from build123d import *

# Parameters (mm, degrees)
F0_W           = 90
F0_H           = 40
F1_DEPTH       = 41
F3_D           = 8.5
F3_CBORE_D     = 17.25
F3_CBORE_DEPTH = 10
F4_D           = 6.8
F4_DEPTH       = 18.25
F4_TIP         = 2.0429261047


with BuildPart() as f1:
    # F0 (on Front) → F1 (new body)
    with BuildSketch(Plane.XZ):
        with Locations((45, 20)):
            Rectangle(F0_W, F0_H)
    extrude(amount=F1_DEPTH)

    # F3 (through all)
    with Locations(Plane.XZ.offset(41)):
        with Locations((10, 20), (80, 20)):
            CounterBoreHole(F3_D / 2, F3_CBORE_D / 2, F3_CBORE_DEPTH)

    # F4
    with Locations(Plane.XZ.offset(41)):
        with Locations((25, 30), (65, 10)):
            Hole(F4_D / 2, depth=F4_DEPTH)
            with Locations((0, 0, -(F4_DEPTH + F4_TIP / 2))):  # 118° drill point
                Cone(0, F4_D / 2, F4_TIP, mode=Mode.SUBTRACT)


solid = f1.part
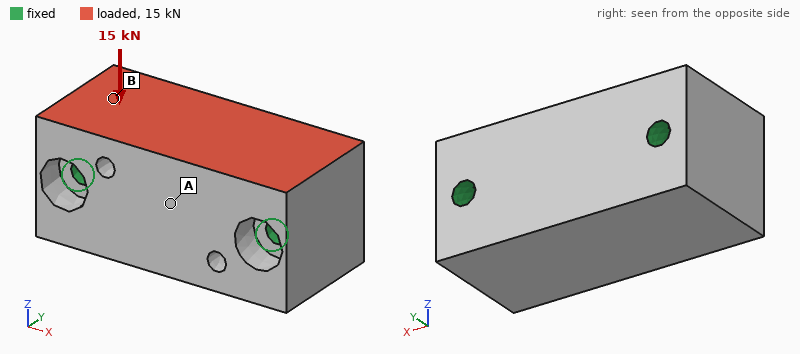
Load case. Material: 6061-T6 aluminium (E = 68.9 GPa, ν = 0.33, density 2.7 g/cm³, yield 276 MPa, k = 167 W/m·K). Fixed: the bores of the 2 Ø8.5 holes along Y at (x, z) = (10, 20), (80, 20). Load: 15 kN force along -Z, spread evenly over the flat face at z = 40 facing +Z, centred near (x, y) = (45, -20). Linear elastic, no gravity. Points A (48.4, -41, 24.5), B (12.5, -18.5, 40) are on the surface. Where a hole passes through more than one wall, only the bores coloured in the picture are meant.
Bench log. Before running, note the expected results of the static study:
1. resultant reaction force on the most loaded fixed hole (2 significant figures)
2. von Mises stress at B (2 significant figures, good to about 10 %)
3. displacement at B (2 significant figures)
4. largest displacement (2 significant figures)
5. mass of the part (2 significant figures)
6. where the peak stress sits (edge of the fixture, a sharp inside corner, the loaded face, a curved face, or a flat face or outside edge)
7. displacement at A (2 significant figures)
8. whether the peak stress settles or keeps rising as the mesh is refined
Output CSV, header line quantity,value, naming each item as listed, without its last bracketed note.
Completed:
quantity,value
resultant reaction force on the most loaded fixed hole,7.5 kN
von Mises stress at B,7.6 MPa
displacement at B,2.9 µm
largest displacement,8.9 µm
mass of the part,370 g
where the peak stress sits,edge of the fixture
displacement at A,7.9 µm
whether the peak stress settles or keeps rising as the mesh is refined,keeps rising
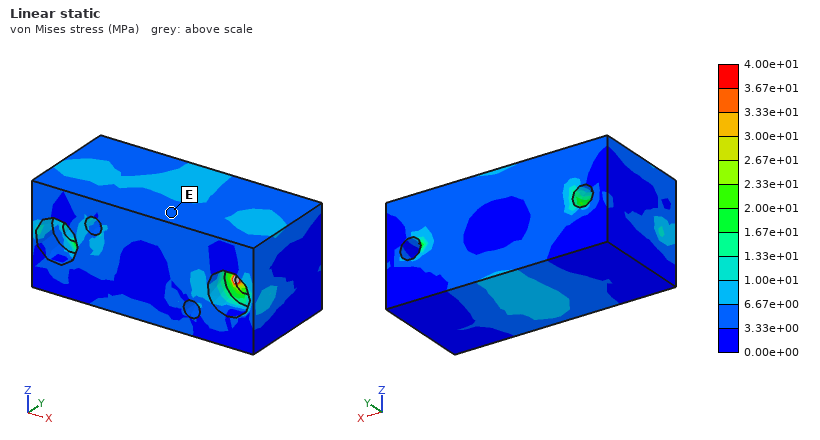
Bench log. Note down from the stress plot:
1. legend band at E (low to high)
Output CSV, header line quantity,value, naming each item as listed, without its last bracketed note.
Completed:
quantity,value
legend band at E,3.33e+00 to 6.67e+00 MPa
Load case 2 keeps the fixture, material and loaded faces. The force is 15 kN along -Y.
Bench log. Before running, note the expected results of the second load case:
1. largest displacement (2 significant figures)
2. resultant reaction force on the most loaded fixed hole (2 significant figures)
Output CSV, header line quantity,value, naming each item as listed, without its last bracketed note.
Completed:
quantity,value
largest displacement,20 µm
resultant reaction force on the most loaded fixed hole,7.6 kN
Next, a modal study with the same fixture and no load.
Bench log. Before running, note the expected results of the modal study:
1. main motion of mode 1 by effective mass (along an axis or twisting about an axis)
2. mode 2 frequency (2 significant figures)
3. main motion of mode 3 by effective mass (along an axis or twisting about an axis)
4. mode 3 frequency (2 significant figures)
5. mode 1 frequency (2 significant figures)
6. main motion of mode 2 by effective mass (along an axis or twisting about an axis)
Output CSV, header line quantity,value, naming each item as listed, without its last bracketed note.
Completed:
quantity,value
main motion of mode 1 by effective mass,along Z
mode 2 frequency,15 kHz
main motion of mode 3 by effective mass,along Z
mode 3 frequency,16 kHz
mode 1 frequency,13 kHz
main motion of mode 2 by effective mass,along Y
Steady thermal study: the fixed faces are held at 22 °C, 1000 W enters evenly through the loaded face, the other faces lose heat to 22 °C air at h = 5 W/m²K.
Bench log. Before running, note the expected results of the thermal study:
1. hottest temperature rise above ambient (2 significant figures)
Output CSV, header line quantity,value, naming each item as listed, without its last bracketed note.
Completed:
quantity,value
hottest temperature rise above ambient,62 K
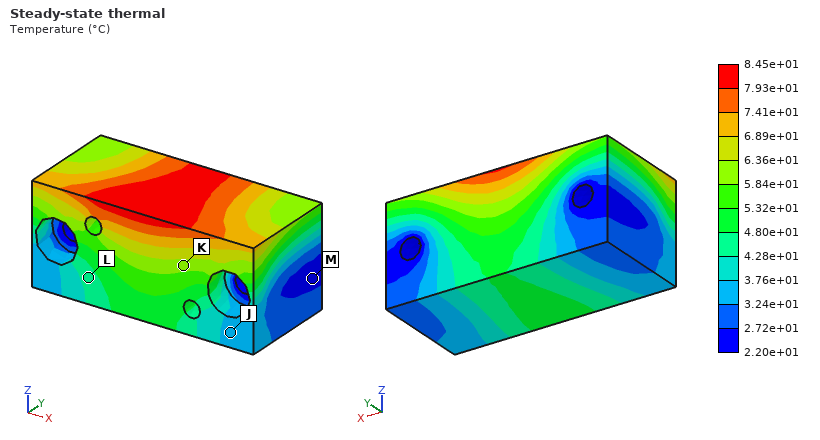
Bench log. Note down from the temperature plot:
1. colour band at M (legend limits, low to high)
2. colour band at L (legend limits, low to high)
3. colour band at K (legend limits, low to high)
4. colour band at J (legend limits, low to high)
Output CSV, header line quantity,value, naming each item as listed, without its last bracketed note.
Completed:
quantity,value
colour band at M,2.20e+01 to 2.72e+01 °C
colour band at L,4.28e+01 to 4.80e+01 °C
colour band at K,5.84e+01 to 6.36e+01 °C
colour band at J,3.24e+01 to 3.76e+01 °C
